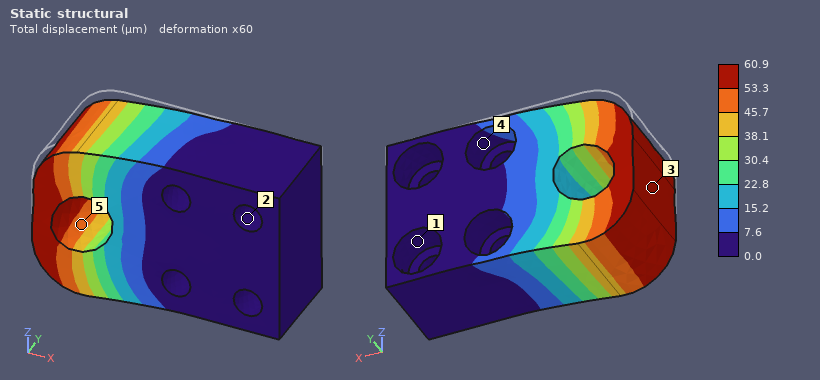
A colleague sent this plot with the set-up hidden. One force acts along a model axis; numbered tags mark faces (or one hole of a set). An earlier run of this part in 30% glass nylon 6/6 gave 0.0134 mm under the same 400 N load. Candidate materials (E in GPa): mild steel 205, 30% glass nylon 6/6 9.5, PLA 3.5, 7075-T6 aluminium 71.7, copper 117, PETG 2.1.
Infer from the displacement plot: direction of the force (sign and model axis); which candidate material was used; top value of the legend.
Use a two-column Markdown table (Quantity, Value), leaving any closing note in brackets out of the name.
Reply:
| Quantity | Value |
|---|---|
| direction of the force | -Z |
| which candidate material was used | PETG |
| top value of the legend | 60.9 µm |
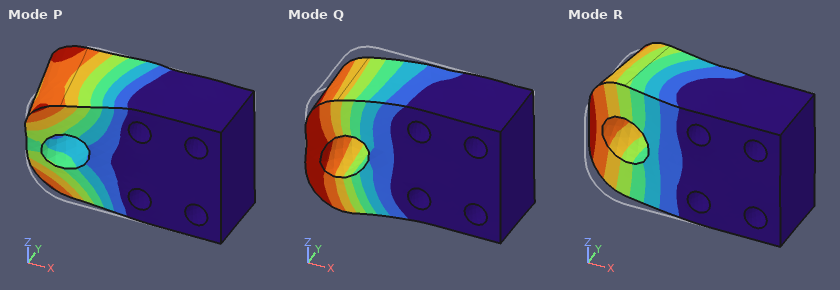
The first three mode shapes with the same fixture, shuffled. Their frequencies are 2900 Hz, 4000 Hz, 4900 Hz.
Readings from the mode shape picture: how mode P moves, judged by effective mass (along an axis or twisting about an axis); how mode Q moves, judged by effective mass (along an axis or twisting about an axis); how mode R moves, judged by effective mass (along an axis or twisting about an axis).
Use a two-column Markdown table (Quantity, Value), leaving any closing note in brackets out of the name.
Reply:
| Quantity | Value |
|---|---|
| how mode P moves, judged by effective mass | twisting about X |
| how mode Q moves, judged by effective mass | along Z |
| how mode R moves, judged by effective mass | along Y |
